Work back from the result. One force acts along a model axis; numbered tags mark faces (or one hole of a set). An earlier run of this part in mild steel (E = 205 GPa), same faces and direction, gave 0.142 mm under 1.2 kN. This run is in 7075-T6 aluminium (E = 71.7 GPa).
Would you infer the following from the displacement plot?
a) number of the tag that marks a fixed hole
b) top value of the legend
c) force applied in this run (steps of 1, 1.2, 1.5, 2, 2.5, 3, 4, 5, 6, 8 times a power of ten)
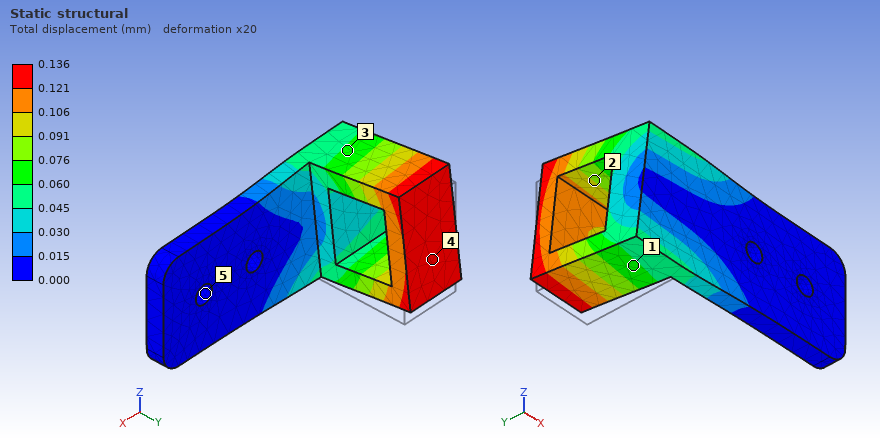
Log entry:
5
0.136 mm
400 N
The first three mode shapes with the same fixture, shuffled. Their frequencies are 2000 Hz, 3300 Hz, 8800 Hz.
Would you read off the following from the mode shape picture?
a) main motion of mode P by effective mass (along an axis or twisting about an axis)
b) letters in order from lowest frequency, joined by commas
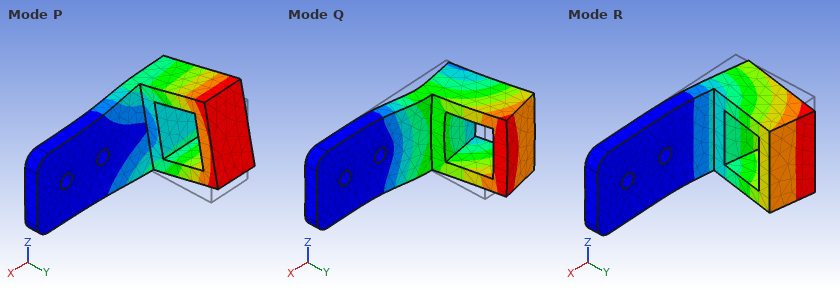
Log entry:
along Z
R, P, Q
